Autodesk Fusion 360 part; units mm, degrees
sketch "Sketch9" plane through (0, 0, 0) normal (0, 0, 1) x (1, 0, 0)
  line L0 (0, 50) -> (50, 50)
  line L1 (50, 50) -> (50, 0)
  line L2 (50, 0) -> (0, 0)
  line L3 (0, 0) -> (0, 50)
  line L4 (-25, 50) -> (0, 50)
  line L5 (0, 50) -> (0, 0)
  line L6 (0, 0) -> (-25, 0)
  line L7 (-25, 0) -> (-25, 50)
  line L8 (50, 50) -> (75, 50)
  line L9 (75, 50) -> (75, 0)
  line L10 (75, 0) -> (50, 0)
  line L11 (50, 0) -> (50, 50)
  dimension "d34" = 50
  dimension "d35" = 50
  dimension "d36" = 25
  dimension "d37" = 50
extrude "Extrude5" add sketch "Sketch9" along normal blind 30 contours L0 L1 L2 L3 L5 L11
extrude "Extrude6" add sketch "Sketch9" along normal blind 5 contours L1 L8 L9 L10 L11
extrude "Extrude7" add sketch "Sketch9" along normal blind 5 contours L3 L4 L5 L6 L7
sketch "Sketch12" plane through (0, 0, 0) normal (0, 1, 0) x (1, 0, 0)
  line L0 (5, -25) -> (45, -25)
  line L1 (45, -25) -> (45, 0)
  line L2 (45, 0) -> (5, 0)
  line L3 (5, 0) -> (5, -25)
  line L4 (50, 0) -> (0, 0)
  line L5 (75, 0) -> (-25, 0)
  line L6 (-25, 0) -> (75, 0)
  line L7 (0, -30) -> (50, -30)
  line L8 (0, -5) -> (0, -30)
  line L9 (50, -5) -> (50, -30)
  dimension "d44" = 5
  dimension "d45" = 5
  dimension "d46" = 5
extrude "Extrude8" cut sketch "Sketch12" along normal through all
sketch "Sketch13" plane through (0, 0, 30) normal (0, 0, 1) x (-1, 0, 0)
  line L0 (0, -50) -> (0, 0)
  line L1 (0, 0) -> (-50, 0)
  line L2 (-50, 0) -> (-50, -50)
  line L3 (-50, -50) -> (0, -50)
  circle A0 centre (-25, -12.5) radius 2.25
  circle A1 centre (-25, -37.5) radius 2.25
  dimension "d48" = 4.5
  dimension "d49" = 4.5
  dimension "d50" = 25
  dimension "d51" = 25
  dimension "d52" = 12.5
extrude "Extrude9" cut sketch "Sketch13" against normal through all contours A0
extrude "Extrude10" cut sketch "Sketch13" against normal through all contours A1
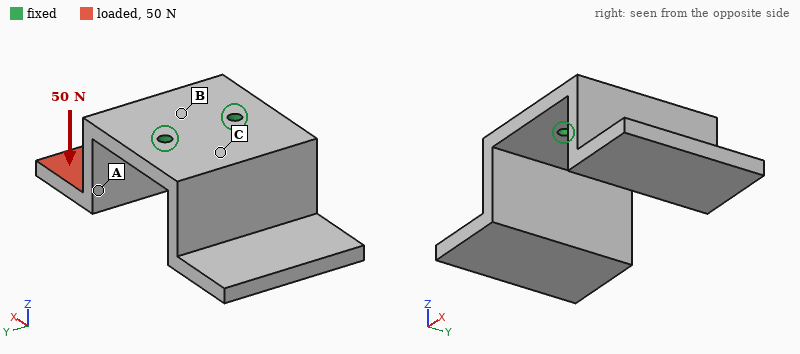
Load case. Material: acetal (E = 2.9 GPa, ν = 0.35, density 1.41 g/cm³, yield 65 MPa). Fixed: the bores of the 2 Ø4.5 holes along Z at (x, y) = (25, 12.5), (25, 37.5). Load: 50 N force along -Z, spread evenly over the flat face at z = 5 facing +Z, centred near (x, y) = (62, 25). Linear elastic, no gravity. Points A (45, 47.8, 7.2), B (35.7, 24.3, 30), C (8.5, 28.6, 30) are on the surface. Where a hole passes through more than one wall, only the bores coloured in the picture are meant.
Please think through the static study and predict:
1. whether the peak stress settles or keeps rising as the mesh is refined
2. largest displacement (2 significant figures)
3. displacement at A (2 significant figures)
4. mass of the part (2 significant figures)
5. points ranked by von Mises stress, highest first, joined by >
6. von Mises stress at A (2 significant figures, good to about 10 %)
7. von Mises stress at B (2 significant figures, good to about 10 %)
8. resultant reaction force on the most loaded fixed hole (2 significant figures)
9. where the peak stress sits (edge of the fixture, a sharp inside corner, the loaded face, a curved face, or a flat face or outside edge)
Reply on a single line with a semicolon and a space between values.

keeps rising; 1.3 mm; 0.50 mm; 53 g; B > A > C; 3.0 MPa; 5.5 MPa; 25 N; edge of the fixture
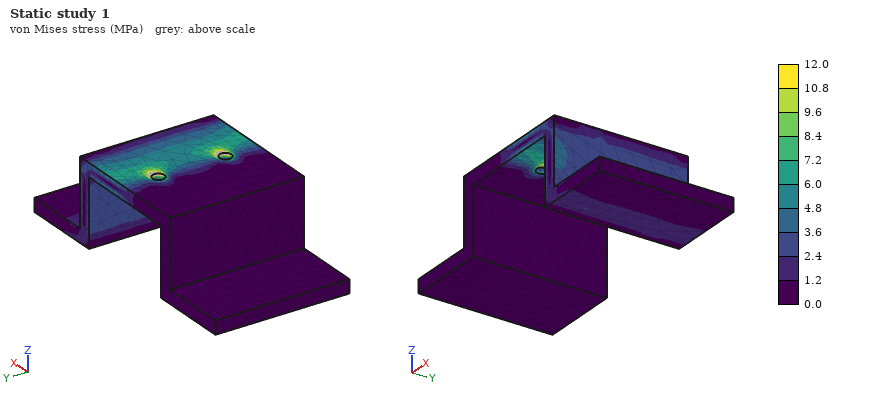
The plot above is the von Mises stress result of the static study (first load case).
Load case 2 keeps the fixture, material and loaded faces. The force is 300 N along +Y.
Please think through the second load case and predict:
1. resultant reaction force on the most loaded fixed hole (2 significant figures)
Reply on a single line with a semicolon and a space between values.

480 N
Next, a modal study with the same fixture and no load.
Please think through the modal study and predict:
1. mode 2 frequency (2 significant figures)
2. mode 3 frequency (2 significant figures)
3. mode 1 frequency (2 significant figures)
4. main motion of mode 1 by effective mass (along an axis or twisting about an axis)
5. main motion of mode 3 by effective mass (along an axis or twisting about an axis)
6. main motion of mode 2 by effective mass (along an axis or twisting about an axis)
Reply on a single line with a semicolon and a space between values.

310 Hz; 680 Hz; 280 Hz; along X; twisting about Z; along Z
